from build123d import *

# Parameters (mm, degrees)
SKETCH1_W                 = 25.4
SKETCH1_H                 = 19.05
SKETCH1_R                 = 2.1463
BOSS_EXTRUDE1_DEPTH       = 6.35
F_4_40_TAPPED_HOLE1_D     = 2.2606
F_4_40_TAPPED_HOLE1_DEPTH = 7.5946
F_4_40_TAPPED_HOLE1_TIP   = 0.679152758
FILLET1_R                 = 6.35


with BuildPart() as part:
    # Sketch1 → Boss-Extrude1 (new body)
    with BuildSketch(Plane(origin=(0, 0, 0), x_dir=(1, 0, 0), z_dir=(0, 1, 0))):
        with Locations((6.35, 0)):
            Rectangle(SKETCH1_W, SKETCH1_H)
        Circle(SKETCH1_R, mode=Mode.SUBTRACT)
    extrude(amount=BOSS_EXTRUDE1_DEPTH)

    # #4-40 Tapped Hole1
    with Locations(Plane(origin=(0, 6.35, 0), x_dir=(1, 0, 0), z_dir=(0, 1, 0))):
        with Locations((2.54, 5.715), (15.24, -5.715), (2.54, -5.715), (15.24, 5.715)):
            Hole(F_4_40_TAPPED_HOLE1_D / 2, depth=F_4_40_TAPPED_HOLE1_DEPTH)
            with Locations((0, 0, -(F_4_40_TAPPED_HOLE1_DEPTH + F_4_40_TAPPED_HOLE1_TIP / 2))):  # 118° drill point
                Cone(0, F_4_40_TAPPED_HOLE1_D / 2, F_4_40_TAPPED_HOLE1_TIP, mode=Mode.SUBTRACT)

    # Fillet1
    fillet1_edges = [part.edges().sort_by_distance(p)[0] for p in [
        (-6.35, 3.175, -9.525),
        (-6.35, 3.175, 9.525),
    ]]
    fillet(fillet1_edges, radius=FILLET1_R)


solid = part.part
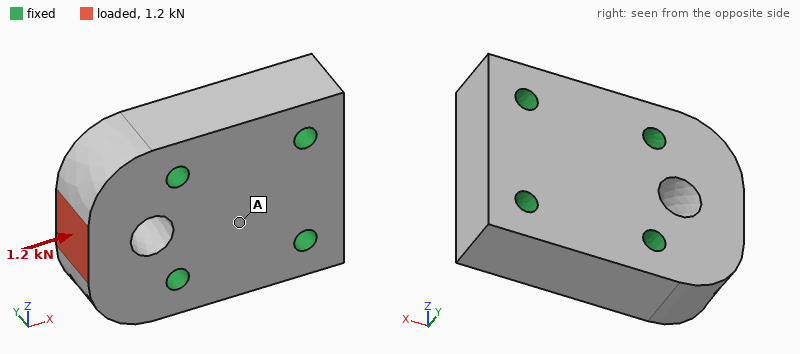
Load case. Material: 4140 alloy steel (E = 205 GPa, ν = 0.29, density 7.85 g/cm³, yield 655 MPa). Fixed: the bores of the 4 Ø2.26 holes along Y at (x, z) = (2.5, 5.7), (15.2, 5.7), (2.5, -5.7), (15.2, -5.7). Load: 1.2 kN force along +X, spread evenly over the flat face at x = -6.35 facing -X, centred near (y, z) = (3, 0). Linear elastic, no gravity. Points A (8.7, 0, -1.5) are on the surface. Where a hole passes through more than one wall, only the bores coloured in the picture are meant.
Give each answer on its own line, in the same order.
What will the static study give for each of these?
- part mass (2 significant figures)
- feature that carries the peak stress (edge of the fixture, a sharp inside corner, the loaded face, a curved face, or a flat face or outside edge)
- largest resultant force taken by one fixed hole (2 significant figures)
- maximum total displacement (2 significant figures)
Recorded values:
22 g
a curved face
610 N
1.5 µm
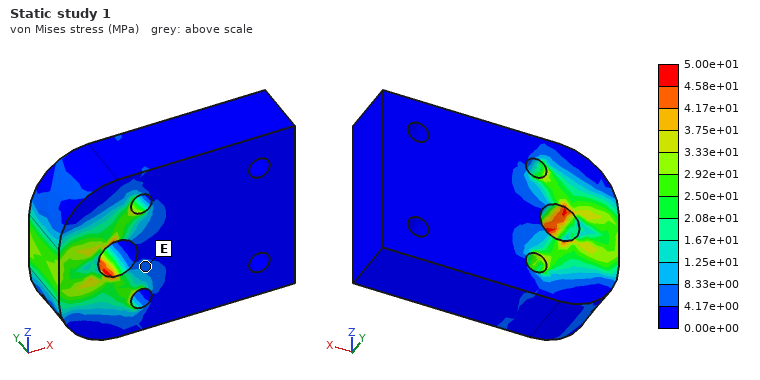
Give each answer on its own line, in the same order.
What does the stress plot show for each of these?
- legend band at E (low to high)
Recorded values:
4.17e+00 to 8.33e+00 MPa
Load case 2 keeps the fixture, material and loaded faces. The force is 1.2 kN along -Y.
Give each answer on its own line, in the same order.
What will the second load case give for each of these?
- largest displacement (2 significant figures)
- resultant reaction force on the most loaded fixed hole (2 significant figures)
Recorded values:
9.3 µm
670 N
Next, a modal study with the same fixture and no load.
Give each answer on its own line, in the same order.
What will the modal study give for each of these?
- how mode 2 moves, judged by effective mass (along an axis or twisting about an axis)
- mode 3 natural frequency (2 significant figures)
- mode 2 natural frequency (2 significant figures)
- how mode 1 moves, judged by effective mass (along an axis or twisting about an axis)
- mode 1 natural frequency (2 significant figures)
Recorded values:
along Z
79 kHz
70 kHz
along Y
50 kHz
